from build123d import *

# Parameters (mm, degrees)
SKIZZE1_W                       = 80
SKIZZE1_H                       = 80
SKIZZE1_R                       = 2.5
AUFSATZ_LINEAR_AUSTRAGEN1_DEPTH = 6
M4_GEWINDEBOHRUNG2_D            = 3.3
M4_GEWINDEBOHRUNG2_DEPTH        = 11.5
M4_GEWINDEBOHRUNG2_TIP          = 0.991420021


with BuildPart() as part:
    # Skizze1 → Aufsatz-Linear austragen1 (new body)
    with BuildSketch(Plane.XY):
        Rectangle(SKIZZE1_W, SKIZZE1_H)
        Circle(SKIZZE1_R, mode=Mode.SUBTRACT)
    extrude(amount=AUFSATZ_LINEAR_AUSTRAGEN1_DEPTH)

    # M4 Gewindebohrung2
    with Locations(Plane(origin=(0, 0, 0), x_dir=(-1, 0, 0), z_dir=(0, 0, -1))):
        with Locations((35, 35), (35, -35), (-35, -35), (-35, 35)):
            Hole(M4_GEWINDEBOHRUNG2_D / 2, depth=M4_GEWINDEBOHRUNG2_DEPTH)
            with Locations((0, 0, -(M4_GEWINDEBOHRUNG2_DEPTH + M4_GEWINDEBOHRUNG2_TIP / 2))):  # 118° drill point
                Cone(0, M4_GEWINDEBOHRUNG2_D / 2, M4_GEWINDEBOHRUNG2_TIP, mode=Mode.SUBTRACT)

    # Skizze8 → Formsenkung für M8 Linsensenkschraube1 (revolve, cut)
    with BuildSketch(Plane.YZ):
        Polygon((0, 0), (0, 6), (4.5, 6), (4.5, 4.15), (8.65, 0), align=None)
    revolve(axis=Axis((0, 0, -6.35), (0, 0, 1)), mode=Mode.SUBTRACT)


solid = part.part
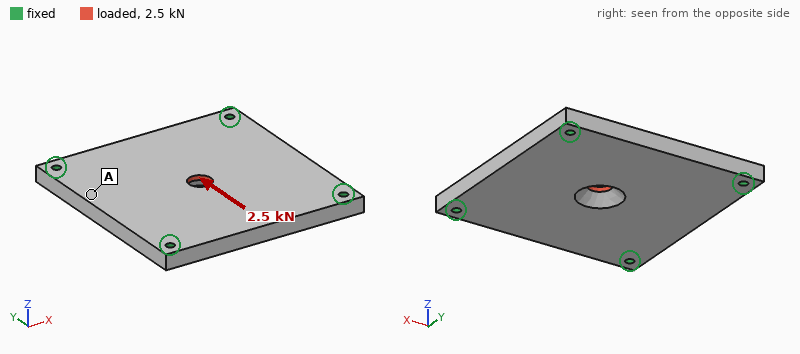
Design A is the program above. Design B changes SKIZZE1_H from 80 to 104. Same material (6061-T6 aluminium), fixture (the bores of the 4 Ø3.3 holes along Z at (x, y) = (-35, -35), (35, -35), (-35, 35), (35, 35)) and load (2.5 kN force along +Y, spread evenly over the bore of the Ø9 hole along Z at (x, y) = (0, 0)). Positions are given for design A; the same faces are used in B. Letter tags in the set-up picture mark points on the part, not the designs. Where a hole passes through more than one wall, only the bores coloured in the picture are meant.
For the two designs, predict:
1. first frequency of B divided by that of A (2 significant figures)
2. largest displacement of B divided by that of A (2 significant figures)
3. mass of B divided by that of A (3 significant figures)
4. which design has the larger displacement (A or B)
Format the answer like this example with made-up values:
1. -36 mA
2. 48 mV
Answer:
1. 1.0
2. 0.92
3. 1.31
4. A
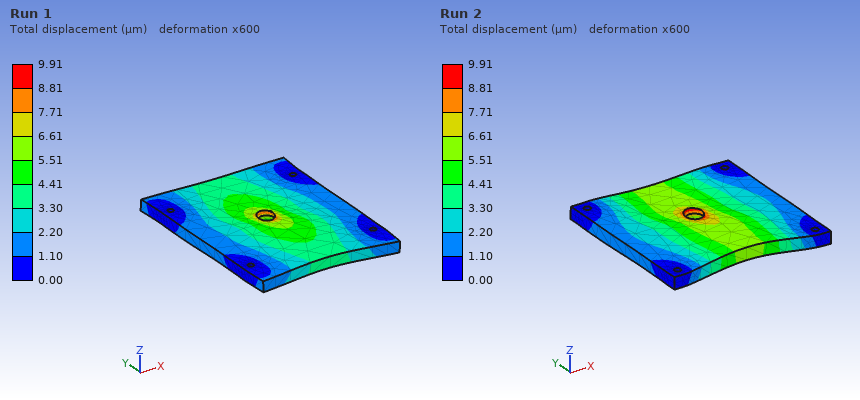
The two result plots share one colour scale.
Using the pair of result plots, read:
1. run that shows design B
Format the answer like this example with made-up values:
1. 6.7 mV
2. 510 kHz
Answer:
1. Run 1
